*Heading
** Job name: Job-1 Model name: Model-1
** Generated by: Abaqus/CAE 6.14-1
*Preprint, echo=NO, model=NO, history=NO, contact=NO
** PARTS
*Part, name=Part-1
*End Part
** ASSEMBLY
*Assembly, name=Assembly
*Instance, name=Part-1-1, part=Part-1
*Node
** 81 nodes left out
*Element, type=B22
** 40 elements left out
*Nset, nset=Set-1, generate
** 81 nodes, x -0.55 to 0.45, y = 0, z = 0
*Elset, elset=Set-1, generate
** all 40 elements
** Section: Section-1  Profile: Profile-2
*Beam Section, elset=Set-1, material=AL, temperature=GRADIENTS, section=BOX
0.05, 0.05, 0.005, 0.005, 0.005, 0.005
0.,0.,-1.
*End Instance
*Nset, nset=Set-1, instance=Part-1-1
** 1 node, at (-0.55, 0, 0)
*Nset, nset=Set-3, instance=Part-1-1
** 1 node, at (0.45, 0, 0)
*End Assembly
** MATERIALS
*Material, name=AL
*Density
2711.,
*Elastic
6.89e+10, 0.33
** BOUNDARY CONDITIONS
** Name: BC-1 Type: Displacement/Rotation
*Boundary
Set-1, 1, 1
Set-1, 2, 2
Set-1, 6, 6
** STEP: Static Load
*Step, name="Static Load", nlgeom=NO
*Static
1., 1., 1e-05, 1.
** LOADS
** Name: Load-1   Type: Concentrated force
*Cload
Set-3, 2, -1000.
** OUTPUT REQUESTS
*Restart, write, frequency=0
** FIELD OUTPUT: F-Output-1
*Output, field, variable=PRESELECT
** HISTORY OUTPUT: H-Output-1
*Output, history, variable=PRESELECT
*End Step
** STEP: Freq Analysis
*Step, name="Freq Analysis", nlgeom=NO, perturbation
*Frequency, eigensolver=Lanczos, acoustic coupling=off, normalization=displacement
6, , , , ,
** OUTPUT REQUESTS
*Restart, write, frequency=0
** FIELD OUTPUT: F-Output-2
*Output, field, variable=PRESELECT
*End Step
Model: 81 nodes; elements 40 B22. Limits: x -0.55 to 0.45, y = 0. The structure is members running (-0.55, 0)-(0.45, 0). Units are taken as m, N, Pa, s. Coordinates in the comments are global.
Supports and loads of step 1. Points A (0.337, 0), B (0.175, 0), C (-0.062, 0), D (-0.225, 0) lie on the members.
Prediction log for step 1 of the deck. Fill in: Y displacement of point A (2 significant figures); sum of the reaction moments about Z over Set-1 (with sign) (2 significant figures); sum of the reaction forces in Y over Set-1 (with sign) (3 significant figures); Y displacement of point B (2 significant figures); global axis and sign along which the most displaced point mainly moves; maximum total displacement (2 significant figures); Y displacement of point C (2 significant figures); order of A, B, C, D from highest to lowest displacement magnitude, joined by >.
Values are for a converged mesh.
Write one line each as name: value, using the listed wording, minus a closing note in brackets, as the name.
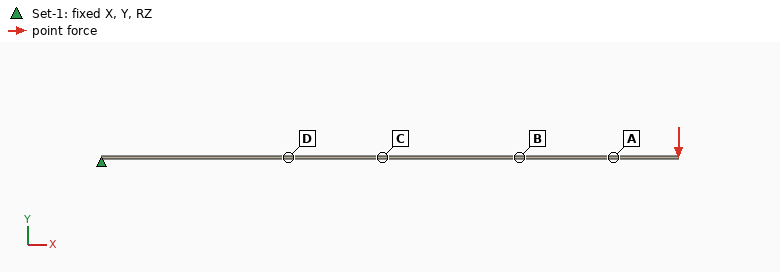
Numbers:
Y displacement of point A: -0.013 m
sum of the reaction moments about Z over Set-1 (with sign): 1000 N·m
sum of the reaction forces in Y over Set-1 (with sign): 1000 N
Y displacement of point B: -0.0095 m
global axis and sign along which the most displaced point mainly moves: -Y
maximum total displacement: 0.016 m
Y displacement of point C: -0.0047 m
order of A, B, C, D from highest to lowest displacement magnitude, joined by >: A > B > C > D
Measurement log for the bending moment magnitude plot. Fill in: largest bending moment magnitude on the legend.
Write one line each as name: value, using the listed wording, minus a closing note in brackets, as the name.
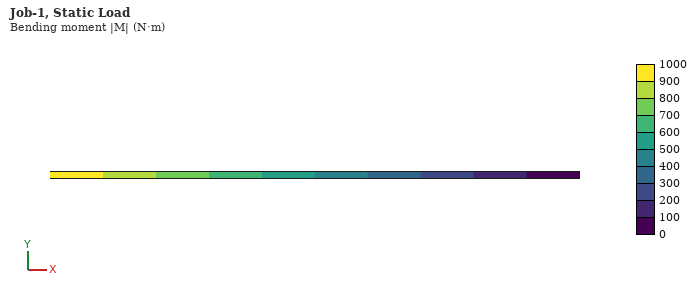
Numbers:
largest bending moment magnitude on the legend: 1000 N·m
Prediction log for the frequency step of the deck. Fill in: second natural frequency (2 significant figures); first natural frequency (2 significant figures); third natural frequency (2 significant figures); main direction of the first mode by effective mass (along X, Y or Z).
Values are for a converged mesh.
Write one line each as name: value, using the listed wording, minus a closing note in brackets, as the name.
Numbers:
second natural frequency: 320 Hz
first natural frequency: 52 Hz
third natural frequency: 850 Hz
main direction of the first mode by effective mass: along Y
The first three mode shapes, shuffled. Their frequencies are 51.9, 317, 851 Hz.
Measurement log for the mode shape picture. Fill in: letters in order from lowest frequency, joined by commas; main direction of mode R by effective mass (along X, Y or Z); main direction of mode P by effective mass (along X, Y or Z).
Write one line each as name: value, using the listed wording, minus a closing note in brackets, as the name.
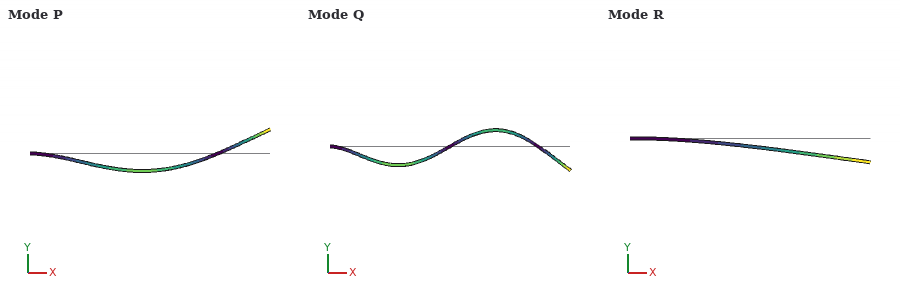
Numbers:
letters in order from lowest frequency, joined by commas: R, P, Q
main direction of mode R by effective mass: along Y
main direction of mode P by effective mass: along Y
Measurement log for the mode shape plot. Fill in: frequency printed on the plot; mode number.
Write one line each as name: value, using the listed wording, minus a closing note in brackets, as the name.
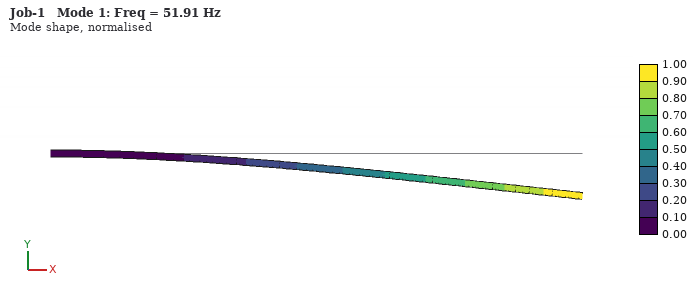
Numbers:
frequency printed on the plot: 51.91 Hz
mode number: 1
